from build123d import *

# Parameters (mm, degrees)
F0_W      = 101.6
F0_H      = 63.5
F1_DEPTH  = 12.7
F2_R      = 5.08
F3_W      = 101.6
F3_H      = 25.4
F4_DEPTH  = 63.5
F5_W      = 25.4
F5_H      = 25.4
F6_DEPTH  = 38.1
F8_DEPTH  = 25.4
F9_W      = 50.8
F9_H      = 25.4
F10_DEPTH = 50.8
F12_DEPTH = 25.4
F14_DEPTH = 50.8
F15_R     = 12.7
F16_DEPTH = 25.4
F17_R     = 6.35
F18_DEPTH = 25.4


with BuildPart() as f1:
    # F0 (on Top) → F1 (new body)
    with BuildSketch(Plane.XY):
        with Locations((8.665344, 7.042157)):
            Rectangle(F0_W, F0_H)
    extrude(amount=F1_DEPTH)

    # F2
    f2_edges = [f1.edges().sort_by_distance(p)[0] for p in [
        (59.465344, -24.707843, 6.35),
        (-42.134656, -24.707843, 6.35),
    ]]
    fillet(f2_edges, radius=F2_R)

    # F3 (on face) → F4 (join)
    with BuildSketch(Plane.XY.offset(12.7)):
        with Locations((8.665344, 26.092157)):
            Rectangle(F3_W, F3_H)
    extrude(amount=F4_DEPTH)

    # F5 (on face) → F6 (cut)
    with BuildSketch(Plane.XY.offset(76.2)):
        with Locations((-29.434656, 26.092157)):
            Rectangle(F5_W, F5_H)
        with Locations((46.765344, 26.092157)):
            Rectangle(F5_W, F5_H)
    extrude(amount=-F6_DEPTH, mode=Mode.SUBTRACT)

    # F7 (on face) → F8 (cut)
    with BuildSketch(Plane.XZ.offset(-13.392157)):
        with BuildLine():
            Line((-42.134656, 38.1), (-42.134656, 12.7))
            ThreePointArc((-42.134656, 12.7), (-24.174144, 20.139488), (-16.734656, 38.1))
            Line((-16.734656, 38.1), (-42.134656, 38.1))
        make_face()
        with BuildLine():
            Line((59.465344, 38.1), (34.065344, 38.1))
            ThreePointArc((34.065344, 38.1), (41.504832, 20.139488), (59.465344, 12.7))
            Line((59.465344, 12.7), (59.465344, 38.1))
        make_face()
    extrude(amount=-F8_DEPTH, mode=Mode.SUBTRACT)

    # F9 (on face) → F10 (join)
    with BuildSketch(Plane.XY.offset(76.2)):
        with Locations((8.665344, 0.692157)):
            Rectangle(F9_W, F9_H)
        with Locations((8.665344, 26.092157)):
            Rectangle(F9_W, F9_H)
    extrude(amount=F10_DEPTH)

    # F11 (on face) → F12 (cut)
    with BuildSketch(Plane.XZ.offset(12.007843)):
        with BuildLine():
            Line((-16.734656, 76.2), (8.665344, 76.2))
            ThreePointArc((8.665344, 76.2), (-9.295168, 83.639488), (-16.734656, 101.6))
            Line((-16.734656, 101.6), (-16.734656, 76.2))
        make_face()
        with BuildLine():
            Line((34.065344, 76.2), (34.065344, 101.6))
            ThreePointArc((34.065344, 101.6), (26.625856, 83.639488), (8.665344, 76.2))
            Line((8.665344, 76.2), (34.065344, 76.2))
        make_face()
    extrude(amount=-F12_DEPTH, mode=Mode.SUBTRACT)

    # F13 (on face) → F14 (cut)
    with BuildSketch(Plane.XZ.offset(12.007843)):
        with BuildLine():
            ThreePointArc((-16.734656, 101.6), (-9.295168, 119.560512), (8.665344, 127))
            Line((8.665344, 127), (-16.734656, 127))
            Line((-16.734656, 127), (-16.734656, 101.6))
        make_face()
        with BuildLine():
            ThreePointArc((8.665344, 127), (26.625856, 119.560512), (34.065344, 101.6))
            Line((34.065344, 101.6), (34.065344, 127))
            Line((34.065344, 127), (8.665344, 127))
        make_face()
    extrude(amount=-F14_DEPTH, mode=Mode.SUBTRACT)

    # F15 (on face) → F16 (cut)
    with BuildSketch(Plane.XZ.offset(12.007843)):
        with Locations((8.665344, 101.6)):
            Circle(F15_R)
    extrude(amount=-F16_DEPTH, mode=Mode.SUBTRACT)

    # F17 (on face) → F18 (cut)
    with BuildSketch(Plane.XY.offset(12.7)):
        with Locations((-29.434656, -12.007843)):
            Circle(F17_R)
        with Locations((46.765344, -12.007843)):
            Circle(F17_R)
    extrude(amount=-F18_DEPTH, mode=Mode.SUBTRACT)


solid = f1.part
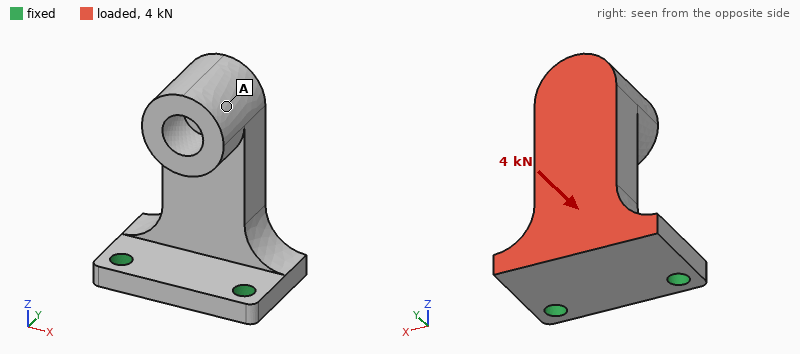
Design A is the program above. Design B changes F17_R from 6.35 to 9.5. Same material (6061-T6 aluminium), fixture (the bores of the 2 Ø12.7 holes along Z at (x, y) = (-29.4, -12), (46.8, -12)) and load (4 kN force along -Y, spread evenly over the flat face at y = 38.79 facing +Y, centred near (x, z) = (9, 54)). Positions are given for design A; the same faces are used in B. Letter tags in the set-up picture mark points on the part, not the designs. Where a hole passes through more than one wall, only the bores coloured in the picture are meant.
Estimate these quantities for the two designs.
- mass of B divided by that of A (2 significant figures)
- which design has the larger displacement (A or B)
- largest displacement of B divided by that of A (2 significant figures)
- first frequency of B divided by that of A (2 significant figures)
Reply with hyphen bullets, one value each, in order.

- 0.98
- A
- 0.87
- 1.1
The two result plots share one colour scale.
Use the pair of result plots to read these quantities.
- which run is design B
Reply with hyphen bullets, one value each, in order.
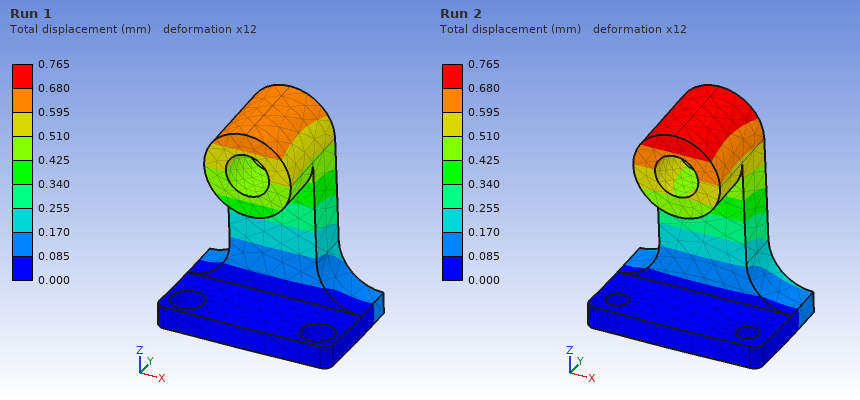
- Run 1
